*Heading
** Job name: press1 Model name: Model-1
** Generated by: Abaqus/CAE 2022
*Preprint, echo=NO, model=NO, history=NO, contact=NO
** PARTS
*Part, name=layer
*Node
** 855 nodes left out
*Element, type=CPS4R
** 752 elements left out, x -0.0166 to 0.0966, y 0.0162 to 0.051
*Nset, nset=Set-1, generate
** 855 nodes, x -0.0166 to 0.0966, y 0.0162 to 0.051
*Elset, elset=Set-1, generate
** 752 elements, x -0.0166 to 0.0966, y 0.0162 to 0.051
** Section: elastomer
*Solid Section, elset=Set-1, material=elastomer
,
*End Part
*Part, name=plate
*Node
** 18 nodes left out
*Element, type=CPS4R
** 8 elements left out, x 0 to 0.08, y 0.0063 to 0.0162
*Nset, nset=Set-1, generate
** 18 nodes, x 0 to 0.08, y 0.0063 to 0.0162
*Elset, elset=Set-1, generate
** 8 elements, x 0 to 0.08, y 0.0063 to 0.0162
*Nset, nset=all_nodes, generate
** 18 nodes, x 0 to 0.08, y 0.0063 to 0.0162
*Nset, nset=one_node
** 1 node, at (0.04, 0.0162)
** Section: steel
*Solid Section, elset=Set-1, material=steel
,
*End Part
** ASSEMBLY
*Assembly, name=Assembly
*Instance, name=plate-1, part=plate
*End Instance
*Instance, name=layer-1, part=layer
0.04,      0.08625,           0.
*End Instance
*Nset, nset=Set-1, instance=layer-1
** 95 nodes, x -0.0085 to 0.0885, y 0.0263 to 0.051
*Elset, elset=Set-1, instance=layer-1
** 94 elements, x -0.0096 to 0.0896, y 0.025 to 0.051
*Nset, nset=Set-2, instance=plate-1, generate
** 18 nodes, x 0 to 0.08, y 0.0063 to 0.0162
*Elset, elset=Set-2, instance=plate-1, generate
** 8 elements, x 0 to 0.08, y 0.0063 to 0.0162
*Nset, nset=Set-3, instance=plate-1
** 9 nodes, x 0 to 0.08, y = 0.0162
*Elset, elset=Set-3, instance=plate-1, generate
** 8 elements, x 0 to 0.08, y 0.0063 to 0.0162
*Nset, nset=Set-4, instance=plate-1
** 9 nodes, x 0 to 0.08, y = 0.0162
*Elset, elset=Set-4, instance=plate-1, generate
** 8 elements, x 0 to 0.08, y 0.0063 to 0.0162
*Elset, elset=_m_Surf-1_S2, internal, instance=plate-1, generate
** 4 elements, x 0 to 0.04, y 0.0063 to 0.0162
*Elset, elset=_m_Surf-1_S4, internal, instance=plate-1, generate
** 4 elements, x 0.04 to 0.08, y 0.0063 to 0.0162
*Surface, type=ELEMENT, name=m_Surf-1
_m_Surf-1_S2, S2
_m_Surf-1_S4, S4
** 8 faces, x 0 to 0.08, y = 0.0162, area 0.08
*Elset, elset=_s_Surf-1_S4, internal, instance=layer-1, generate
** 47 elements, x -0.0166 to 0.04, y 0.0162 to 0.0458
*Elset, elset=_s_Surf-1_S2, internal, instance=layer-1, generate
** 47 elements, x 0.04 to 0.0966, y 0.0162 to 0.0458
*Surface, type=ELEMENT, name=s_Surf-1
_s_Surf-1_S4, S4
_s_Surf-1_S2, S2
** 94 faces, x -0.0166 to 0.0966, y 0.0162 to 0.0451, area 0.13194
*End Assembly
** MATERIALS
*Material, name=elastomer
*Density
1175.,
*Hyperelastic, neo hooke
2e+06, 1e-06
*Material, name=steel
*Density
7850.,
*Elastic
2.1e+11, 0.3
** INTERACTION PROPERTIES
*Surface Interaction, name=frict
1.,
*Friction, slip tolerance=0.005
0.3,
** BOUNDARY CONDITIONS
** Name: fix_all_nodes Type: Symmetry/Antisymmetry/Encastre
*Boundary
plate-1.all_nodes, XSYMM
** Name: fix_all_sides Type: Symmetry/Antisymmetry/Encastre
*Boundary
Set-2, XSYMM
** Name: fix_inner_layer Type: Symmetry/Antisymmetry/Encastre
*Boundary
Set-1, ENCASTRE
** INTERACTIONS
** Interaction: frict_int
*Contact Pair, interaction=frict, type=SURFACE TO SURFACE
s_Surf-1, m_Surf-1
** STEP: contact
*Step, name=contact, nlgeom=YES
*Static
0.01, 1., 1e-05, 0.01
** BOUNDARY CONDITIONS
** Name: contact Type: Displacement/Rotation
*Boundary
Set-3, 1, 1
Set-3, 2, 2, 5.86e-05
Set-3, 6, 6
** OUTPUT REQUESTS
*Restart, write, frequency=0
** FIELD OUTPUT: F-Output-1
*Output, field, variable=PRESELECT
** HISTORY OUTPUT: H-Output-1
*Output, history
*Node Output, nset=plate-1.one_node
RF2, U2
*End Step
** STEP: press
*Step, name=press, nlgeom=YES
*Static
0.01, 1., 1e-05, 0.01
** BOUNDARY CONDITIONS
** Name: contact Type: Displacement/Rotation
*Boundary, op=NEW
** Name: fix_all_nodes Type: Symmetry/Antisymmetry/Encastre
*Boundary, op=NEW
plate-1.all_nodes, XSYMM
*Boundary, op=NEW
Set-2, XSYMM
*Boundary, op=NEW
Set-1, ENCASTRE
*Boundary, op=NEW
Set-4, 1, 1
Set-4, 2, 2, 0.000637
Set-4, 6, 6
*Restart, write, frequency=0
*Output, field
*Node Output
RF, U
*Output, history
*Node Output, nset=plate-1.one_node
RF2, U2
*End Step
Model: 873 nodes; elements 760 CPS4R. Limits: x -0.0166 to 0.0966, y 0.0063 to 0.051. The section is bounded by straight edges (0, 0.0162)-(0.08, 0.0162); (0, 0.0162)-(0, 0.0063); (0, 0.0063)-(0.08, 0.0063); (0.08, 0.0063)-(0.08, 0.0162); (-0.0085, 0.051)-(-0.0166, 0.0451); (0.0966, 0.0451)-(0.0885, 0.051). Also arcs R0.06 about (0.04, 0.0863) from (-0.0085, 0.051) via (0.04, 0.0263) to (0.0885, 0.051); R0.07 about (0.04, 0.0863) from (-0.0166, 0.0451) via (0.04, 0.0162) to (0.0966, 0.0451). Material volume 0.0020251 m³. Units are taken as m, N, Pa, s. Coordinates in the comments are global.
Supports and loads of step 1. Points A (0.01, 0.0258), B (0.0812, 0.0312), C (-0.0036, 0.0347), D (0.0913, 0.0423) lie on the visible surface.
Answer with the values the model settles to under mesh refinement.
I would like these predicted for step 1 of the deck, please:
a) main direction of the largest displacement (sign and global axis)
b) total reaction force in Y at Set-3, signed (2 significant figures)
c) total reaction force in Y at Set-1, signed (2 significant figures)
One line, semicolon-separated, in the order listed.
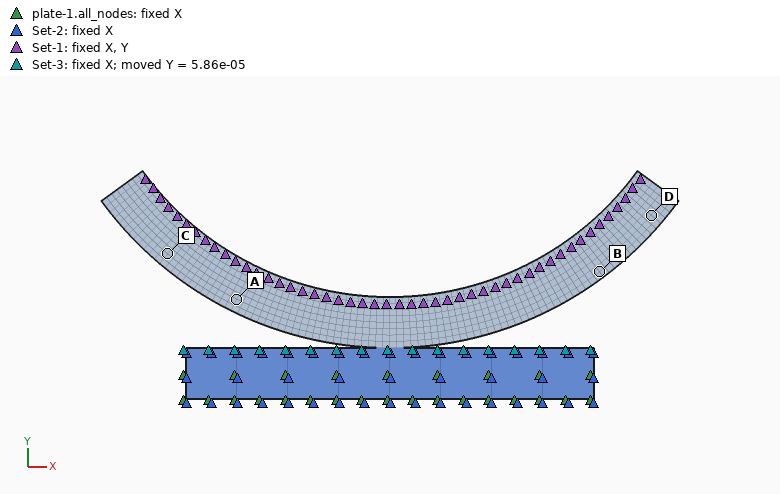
+Y; 19 N; -19 N
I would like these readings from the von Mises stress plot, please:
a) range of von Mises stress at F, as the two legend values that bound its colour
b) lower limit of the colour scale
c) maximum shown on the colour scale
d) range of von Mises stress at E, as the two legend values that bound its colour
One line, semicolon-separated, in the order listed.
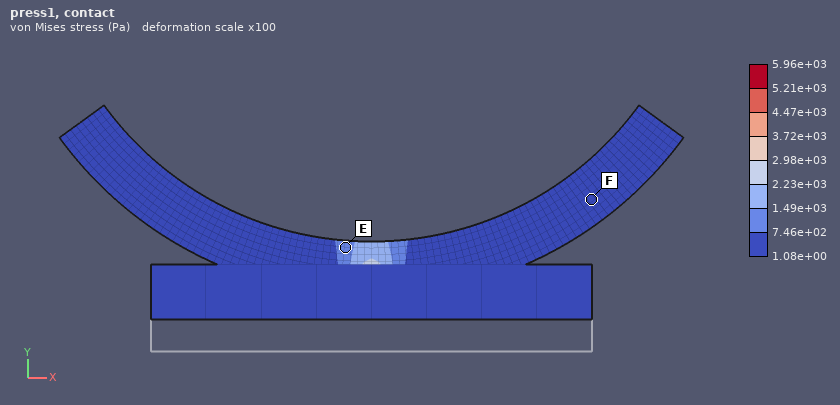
1.08e+00 to 7.46e+02 Pa; 1.08e+00 Pa; 5.96e+03 Pa; 7.46e+02 to 1.49e+03 Pa
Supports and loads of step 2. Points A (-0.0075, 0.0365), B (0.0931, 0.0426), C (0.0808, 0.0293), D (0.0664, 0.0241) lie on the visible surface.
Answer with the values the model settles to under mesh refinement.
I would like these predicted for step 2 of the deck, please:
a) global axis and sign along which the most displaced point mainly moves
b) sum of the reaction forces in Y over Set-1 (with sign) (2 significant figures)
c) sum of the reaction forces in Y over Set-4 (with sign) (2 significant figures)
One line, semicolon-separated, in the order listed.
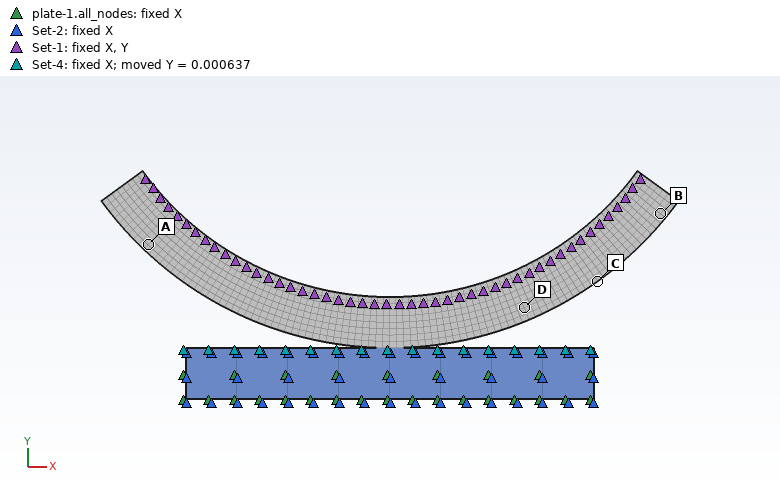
+Y; -700 N; 700 N
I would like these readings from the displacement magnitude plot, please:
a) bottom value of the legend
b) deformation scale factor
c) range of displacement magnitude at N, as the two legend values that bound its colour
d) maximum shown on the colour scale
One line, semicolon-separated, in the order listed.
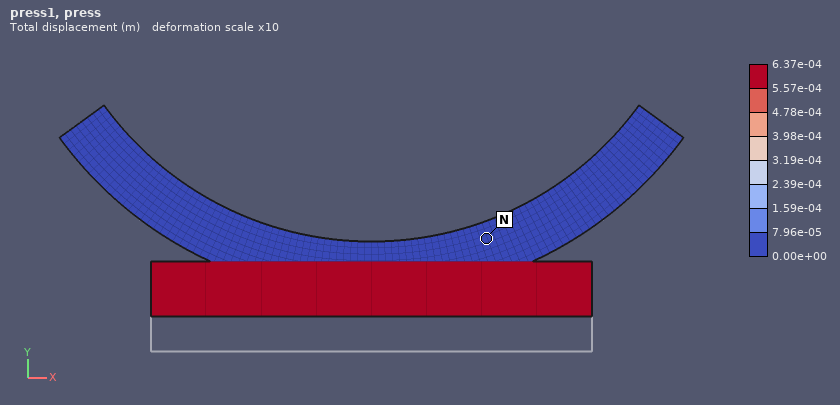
0.00e+00 m; 10; 0.00e+00 to 7.96e-05 m; 6.37e-04 m
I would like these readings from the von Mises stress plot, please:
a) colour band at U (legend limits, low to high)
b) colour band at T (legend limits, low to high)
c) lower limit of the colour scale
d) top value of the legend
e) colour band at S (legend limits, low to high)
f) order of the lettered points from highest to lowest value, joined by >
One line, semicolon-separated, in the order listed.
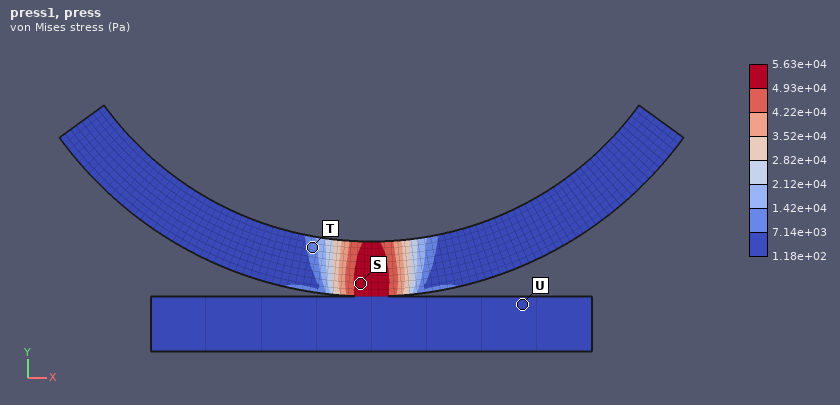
1.18e+02 to 7.14e+03 Pa; 7.14e+03 to 1.42e+04 Pa; 1.18e+02 Pa; 5.63e+04 Pa; 4.93e+04 to 5.63e+04 Pa; S > T > U
